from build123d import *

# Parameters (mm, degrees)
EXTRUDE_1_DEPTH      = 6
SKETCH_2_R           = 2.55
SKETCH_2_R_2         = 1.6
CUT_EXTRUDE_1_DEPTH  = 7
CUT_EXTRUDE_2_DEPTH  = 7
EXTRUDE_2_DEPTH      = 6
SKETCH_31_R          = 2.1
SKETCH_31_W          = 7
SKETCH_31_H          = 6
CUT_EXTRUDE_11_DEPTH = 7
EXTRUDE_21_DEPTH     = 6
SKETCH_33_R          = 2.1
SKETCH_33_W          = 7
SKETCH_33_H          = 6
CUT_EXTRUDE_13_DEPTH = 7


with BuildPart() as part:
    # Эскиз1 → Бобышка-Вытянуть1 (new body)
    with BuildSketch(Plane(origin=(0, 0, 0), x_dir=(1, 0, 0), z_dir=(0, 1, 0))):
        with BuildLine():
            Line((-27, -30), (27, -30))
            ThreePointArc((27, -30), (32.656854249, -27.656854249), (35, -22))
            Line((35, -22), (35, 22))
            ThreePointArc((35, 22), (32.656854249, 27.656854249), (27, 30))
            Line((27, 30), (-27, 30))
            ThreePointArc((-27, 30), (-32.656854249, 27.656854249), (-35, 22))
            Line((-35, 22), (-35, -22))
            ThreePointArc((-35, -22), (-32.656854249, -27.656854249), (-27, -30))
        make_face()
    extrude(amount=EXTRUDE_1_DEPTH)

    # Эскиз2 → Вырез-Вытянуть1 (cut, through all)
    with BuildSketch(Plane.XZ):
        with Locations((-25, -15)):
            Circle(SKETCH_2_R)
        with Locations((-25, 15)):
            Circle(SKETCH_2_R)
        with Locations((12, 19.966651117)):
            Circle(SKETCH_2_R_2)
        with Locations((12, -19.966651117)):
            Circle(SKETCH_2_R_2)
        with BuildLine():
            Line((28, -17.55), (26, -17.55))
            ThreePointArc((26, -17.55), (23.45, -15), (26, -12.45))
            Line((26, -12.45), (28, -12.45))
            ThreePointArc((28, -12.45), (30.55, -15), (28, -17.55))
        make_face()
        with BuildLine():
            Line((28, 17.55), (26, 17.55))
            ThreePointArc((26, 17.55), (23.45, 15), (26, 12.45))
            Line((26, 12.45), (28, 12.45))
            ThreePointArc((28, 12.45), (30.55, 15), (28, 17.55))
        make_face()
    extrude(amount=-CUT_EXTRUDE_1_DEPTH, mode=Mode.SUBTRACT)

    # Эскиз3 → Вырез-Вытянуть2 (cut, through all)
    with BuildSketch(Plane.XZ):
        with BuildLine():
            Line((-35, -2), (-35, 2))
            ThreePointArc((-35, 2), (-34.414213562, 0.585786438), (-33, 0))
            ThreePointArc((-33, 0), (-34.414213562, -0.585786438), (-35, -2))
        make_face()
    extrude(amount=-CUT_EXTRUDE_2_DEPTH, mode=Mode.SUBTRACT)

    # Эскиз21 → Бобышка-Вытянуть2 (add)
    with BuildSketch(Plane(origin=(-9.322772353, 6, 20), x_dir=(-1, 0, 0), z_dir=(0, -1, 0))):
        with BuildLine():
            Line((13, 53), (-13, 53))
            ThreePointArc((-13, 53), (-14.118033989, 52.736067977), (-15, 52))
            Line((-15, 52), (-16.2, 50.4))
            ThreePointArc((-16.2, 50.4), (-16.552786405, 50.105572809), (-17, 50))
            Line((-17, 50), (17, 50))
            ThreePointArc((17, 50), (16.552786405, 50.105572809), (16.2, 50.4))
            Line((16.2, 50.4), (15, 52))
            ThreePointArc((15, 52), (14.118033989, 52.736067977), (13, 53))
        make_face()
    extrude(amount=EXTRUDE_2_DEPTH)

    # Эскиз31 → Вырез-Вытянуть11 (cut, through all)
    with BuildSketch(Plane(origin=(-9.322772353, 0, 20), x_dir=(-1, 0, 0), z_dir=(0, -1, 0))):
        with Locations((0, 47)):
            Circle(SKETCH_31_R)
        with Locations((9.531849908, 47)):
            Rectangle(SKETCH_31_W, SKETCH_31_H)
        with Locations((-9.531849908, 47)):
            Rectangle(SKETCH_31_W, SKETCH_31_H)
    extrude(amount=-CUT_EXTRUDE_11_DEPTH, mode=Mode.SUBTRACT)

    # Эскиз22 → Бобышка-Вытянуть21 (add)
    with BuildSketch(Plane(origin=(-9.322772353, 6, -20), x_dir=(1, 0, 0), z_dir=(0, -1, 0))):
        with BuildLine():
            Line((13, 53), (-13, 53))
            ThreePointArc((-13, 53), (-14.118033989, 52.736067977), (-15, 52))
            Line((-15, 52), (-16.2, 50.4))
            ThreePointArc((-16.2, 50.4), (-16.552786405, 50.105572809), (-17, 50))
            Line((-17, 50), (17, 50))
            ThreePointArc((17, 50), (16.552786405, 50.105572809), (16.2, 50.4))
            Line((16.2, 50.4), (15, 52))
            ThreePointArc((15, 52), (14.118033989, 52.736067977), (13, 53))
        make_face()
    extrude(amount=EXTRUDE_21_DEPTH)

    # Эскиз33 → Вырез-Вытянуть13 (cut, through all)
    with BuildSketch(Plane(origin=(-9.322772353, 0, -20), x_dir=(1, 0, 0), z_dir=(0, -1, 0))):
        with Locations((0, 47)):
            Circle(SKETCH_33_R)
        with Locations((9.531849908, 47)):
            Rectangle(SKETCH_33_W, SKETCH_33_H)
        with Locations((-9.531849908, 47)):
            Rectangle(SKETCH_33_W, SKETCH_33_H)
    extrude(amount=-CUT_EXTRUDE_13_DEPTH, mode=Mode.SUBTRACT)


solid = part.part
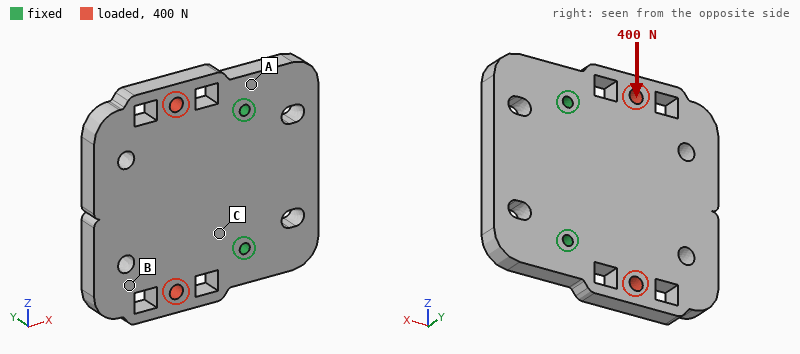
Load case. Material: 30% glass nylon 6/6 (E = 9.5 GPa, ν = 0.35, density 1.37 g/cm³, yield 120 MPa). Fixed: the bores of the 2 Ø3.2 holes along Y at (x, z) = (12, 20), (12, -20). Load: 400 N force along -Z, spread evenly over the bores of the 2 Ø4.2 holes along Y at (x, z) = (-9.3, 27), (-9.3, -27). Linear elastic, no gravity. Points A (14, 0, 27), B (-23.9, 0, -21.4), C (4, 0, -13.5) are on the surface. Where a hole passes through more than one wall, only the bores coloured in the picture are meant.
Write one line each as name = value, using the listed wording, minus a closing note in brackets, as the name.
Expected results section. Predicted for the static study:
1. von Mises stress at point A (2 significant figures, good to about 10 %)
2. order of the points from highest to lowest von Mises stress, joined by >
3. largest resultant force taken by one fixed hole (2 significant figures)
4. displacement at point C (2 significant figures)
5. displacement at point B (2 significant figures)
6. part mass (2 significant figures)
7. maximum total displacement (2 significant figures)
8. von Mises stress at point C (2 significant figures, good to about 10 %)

von Mises stress at point A = 1.4 MPa
order of the points from highest to lowest von Mises stress, joined by > = C > A > B
largest resultant force taken by one fixed hole = 290 N
displacement at point C = 4.6 µm
displacement at point B = 16 µm
part mass = 33 g
maximum total displacement = 18 µm
von Mises stress at point C = 3.0 MPa
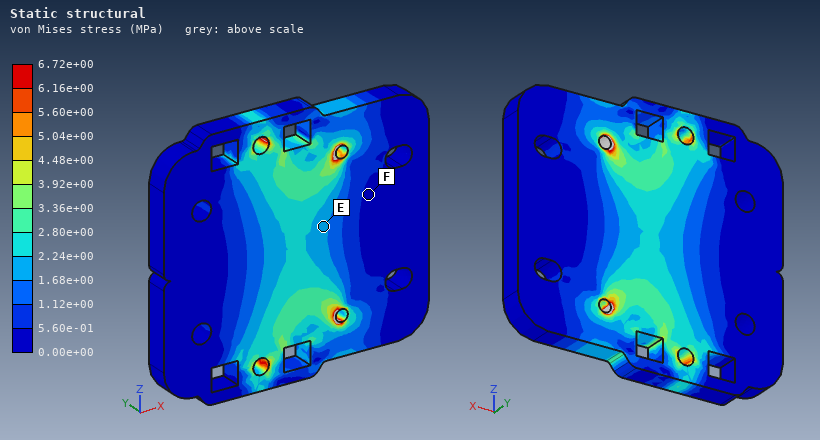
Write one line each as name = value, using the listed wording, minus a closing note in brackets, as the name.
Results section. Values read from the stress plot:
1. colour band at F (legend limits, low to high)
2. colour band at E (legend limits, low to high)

colour band at F = 0.00e+00 to 5.60e-01 MPa
colour band at E = 1.68e+00 to 2.24e+00 MPa
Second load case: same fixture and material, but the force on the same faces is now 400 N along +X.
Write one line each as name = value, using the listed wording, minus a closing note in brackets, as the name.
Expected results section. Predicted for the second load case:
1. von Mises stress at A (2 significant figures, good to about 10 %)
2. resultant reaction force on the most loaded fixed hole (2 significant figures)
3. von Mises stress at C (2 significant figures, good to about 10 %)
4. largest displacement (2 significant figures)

von Mises stress at A = 0.94 MPa
resultant reaction force on the most loaded fixed hole = 200 N
von Mises stress at C = 0.88 MPa
largest displacement = 9.3 µm
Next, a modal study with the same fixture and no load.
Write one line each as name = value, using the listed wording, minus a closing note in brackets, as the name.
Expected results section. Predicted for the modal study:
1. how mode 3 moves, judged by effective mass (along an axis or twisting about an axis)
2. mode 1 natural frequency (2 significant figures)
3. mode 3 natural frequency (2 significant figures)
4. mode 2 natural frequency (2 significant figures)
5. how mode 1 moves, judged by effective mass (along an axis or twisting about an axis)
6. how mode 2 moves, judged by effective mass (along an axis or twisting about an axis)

how mode 3 moves, judged by effective mass = along Y
mode 1 natural frequency = 990 Hz
mode 3 natural frequency = 3800 Hz
mode 2 natural frequency = 2200 Hz
how mode 1 moves, judged by effective mass = along Y
how mode 2 moves, judged by effective mass = twisting about X
